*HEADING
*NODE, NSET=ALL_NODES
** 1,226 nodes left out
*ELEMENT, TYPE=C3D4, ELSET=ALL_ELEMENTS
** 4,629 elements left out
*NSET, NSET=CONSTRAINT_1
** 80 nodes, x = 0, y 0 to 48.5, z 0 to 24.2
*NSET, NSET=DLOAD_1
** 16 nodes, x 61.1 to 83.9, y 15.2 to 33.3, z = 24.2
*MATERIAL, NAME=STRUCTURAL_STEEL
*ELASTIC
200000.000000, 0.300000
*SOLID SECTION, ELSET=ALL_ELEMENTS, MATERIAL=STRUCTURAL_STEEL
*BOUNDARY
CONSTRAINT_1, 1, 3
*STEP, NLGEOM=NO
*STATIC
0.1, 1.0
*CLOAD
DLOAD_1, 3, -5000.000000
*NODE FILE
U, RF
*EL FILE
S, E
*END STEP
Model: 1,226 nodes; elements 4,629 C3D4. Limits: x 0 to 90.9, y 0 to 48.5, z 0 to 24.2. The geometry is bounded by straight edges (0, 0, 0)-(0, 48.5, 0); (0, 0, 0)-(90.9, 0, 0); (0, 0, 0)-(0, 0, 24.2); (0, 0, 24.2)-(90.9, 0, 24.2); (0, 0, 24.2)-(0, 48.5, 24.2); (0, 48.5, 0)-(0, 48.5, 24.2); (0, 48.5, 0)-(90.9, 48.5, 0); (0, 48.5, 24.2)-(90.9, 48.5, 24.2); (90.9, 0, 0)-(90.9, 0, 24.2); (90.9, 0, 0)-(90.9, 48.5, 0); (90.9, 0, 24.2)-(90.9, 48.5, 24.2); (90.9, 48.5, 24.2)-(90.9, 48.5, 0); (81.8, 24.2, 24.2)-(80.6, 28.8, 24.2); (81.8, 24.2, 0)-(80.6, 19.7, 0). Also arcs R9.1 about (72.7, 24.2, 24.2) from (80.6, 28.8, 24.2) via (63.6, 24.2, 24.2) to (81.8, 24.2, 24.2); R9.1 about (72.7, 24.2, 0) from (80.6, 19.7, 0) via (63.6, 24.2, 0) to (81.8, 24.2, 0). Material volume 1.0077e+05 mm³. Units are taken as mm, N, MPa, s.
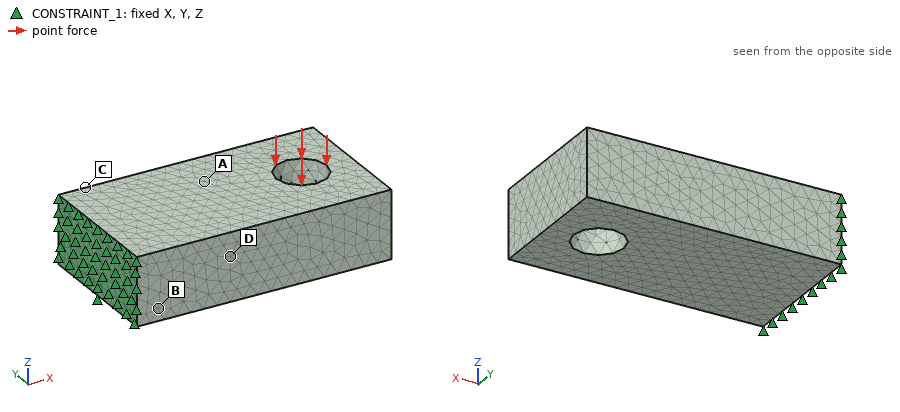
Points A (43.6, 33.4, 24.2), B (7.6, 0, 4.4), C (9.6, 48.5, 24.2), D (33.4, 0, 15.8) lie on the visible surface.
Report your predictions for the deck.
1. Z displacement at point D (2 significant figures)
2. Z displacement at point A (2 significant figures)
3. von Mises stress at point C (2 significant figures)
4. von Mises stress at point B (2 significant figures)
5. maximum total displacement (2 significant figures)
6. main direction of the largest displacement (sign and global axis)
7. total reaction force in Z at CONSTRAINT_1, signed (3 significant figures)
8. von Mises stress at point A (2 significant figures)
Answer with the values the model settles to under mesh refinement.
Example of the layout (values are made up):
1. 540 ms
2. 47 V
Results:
1. -0.24 mm
2. -0.42 mm
3. 980 MPa
4. 630 MPa
5. 1.3 mm
6. -Z
7. 80000 N
8. 490 MPa
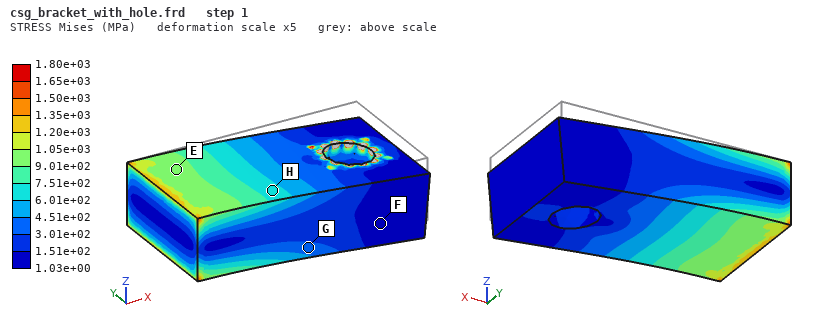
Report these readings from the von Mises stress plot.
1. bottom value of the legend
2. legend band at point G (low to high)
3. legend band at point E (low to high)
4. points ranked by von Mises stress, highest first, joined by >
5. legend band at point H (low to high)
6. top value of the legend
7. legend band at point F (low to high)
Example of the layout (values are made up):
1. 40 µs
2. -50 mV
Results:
1. 1.03e+00 MPa
2. 3.01e+02 to 4.51e+02 MPa
3. 9.01e+02 to 1.05e+03 MPa
4. E > H > G > F
5. 6.01e+02 to 7.51e+02 MPa
6. 1.80e+03 MPa
7. 1.03e+00 to 1.51e+02 MPa
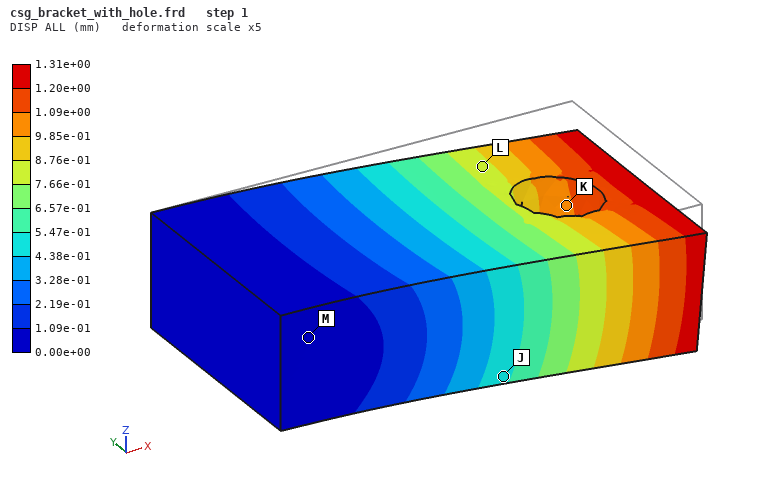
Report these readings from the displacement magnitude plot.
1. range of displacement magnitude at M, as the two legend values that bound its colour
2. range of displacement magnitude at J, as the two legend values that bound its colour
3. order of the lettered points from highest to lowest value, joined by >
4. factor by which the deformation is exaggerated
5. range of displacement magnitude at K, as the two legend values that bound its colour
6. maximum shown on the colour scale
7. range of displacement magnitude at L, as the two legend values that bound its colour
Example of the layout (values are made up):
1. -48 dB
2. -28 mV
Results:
1. 0.00e+00 to 1.09e-01 mm
2. 4.38e-01 to 5.47e-01 mm
3. K > L > J > M
4. 5
5. 9.85e-01 to 1.09e+00 mm
6. 1.31e+00 mm
7. 7.66e-01 to 8.76e-01 mm
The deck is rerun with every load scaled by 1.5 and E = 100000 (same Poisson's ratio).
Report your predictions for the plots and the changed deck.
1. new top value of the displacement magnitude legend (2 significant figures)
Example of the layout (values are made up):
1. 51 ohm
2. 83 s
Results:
1. 3.9 mm
